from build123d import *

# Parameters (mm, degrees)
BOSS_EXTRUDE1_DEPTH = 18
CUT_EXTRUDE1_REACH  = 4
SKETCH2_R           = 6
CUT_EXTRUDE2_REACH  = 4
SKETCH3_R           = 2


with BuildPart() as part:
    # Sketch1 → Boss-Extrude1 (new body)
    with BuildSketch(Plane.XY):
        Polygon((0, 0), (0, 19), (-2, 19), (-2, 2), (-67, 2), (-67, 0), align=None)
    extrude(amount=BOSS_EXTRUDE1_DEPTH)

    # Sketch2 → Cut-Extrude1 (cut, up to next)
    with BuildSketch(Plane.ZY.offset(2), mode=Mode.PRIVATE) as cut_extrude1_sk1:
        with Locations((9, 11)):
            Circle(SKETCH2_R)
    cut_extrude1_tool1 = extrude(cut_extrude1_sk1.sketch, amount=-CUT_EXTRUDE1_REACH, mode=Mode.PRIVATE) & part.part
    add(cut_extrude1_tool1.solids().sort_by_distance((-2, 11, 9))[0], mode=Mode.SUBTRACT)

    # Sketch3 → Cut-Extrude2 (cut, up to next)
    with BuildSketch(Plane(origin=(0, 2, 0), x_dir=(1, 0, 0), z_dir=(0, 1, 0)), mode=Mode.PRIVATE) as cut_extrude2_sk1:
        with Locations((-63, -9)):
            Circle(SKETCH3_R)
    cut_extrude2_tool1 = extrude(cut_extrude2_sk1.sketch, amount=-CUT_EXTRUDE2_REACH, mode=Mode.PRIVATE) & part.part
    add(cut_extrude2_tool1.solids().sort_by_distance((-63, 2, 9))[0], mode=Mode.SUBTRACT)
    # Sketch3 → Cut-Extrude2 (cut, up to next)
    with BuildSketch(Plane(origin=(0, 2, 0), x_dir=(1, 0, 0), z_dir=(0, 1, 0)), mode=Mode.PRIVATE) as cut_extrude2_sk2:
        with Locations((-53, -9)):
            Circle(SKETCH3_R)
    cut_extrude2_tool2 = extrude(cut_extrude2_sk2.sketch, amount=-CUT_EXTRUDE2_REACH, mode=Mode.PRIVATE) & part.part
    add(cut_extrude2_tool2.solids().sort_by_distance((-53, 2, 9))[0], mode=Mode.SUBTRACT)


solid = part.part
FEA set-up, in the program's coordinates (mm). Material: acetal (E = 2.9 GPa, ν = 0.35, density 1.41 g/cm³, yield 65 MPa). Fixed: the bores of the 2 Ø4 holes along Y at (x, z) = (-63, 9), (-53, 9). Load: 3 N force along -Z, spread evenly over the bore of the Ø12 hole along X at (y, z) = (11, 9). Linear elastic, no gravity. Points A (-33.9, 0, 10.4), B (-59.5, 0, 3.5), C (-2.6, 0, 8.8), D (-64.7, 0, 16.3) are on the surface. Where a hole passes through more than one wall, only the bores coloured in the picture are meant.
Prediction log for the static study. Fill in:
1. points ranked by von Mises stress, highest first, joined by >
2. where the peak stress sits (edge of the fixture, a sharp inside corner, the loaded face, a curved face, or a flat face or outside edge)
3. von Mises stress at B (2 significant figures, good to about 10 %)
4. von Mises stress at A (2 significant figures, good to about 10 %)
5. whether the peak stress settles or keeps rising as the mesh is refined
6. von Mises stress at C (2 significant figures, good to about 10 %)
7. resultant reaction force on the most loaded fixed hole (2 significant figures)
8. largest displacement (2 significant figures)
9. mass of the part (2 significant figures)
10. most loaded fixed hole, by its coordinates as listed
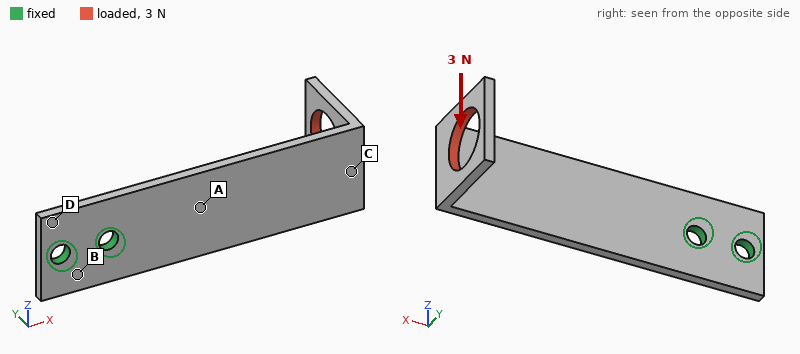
A > C > B > D
edge of the fixture
0.94 MPa
2.1 MPa
keeps rising
1.3 MPa
12 N
0.68 mm
3.9 g
(-53, 9)
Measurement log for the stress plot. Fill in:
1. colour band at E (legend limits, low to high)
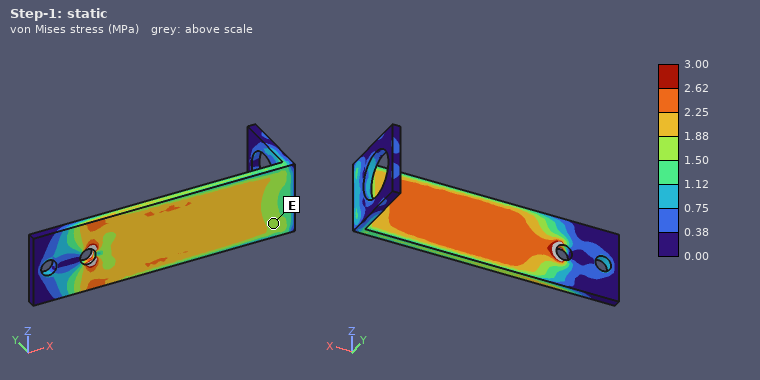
1.50 to 1.88 MPa
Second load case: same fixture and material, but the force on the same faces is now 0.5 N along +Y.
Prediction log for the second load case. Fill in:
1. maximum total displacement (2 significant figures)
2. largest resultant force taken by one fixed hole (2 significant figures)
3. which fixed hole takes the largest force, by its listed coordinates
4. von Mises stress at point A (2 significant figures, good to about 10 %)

0.73 mm
1.0 N
(-53, 9)
1.3 MPa
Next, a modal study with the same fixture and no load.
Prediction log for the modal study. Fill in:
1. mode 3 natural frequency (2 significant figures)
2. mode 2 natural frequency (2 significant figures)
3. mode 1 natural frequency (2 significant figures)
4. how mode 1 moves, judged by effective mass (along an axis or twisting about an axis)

660 Hz
460 Hz
130 Hz
along Y
